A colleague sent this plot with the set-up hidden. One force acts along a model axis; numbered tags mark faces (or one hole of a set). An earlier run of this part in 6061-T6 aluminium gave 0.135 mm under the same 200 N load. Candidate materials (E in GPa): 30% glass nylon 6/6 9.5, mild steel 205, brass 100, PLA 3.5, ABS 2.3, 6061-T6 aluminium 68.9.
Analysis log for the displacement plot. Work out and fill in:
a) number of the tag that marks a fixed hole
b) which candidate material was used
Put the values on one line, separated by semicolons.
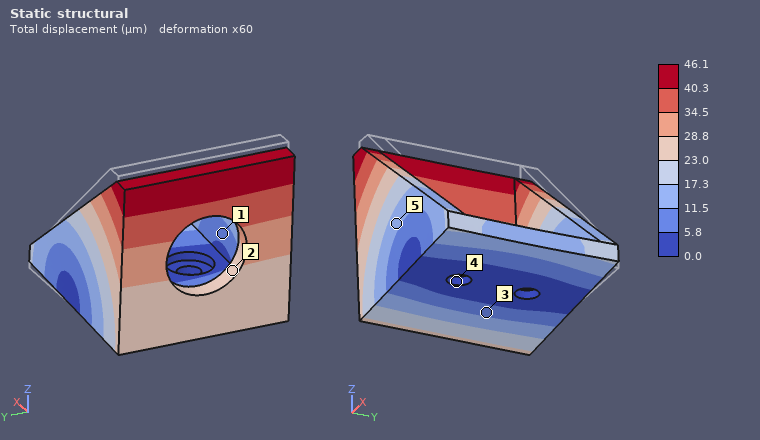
4; mild steel
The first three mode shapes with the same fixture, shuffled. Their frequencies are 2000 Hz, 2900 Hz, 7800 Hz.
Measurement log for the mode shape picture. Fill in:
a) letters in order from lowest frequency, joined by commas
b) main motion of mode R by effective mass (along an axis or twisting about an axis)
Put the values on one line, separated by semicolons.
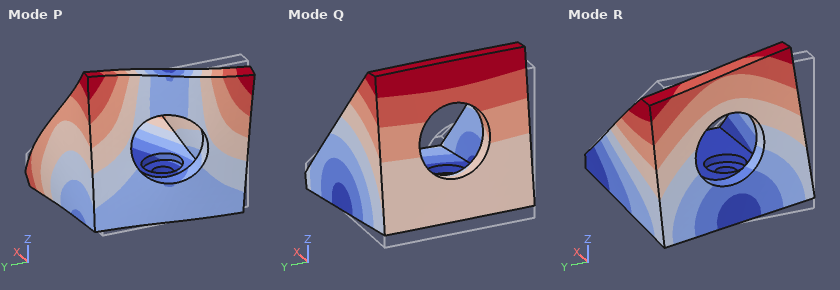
Q, R, P; along Y
